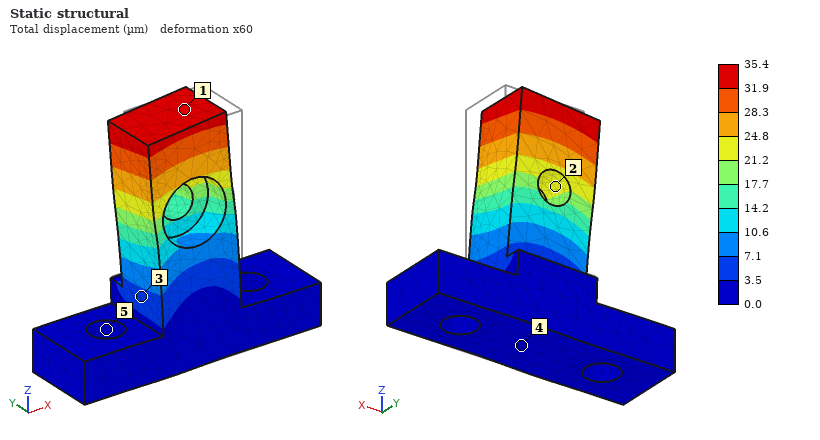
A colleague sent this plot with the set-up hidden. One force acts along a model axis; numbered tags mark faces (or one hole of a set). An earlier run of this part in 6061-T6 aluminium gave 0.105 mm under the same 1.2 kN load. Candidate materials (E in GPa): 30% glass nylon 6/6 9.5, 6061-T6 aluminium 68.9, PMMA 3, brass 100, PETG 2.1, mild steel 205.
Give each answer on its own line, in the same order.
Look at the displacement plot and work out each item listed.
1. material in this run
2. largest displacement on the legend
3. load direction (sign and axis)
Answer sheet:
mild steel
35.4 µm
-X
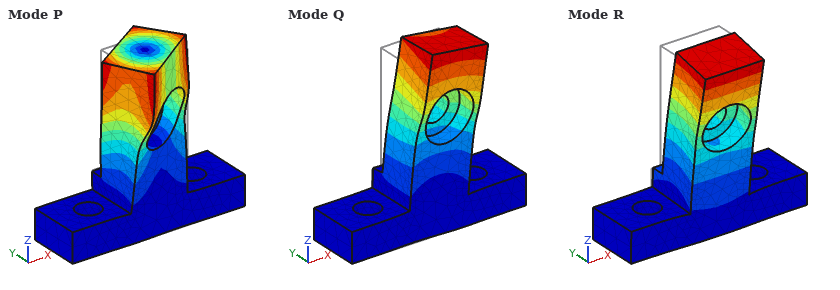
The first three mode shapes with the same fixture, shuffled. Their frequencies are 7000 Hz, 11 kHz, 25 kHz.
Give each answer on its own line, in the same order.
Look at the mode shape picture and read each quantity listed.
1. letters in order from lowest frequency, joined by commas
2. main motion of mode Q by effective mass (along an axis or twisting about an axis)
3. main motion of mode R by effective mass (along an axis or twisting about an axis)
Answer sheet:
R, Q, P
along X
along Y
